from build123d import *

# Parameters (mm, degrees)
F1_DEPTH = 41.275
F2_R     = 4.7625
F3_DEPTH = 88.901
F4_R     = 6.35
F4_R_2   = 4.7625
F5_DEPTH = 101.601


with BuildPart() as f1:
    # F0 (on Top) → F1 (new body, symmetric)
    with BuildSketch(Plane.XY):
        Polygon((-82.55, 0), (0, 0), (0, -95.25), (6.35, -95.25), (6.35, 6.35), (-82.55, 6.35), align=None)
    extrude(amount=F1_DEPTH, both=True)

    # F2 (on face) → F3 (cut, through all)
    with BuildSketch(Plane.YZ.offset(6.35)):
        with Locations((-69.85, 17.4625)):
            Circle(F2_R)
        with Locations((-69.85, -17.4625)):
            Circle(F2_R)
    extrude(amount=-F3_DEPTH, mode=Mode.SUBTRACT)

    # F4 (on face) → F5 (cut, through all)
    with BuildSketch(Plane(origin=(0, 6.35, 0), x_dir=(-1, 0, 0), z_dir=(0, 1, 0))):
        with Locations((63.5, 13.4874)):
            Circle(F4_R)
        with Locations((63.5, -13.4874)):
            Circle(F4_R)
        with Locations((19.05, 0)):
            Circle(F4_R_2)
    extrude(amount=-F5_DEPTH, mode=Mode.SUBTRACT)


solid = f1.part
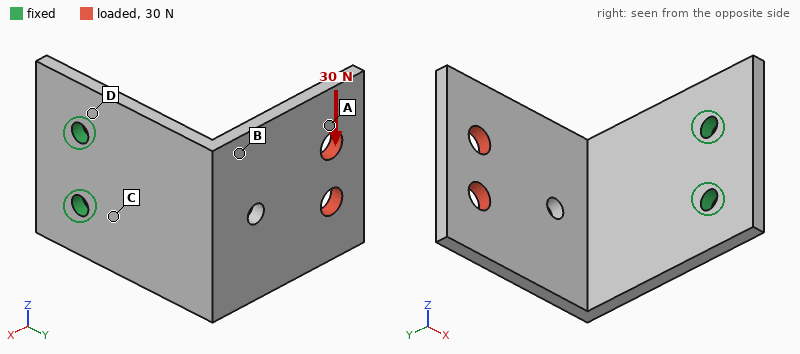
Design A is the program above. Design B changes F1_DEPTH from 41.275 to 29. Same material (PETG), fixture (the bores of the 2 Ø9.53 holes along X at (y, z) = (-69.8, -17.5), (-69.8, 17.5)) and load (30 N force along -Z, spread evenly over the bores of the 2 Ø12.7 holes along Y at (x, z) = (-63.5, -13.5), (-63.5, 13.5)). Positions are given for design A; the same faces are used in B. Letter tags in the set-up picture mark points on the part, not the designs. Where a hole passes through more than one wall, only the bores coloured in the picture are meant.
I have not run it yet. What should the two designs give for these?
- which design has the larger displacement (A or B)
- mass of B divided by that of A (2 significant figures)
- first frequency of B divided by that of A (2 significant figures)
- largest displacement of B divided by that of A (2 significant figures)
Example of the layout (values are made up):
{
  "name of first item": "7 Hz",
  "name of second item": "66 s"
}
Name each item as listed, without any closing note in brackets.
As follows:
{
  "which design has the larger displacement": "B",
  "mass of B divided by that of A": "0.69",
  "first frequency of B divided by that of A": "1.0",
  "largest displacement of B divided by that of A": "1.5"
}
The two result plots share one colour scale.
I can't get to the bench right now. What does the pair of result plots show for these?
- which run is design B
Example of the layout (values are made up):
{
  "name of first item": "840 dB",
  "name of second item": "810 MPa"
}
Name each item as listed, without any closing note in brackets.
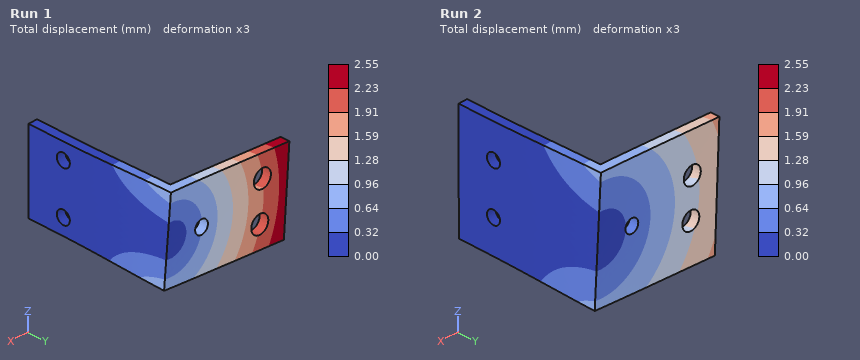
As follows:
{
  "which run is design B": "Run 1"
}
